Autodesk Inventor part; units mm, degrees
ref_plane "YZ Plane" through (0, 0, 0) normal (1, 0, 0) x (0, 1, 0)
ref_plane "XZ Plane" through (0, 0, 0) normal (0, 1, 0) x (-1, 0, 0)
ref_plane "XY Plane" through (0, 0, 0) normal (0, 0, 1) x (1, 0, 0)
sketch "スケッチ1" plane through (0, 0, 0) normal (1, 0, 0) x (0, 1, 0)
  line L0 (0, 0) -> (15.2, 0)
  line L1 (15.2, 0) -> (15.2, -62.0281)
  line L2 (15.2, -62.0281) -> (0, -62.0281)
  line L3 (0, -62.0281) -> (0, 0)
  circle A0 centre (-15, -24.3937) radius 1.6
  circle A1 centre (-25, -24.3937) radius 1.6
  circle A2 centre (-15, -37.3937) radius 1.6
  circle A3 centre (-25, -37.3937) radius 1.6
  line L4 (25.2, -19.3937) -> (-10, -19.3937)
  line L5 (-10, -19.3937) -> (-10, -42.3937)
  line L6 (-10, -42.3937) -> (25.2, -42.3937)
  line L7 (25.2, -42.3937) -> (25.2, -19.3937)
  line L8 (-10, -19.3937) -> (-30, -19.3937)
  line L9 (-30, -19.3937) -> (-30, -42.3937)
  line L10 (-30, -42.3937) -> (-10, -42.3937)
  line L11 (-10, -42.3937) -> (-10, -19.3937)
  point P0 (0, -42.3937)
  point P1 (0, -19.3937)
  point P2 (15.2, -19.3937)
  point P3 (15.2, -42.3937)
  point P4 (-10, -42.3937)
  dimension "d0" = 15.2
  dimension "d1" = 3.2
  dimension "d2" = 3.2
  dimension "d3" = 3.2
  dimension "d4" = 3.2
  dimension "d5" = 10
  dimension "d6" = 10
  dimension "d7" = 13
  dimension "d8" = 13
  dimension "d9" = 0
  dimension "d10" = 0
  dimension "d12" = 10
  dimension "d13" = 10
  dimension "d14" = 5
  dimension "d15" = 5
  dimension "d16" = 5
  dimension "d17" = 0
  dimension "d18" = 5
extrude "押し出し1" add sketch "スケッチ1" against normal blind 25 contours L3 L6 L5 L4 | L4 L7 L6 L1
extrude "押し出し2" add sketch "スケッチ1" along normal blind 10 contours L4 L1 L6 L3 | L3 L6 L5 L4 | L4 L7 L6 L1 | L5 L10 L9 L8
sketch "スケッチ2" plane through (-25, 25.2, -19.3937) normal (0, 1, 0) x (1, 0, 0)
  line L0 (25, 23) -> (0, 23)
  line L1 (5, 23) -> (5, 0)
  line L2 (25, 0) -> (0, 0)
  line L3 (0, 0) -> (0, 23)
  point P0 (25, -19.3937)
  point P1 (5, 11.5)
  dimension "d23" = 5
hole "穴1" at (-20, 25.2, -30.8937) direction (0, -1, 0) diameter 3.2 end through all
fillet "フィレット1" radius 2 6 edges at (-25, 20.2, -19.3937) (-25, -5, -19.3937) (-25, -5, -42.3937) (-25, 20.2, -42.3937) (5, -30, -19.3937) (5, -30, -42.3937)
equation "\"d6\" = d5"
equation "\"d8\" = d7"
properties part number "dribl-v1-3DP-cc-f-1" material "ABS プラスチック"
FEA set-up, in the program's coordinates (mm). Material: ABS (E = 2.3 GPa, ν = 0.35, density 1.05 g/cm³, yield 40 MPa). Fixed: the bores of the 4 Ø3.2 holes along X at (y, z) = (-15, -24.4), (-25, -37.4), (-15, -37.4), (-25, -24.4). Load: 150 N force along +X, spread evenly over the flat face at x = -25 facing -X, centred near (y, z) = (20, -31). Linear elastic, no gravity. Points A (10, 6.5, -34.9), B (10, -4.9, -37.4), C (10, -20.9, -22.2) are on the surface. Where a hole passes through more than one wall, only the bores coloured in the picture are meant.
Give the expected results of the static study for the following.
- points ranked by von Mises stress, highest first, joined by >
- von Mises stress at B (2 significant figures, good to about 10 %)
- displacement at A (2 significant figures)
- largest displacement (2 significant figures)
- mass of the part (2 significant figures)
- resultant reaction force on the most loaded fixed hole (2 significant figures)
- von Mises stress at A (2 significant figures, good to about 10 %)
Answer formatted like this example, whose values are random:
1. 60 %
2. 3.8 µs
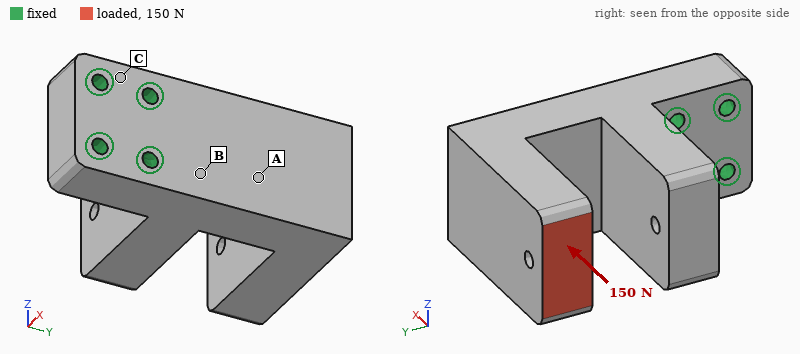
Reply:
1. B > A > C
2. 7.7 MPa
3. 0.23 mm
4. 0.79 mm
5. 25 g
6. 110 N
7. 4.8 MPa
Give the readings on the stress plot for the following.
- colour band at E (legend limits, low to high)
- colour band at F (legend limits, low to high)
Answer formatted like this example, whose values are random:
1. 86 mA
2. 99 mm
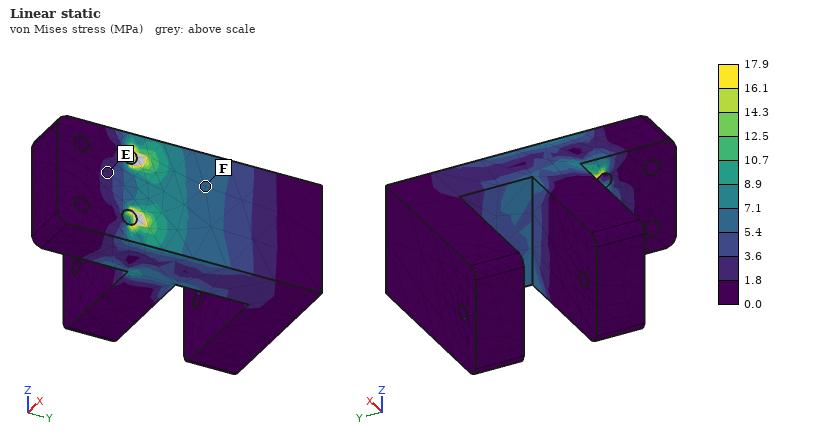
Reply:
1. 1.8 to 3.6 MPa
2. 5.4 to 7.1 MPa
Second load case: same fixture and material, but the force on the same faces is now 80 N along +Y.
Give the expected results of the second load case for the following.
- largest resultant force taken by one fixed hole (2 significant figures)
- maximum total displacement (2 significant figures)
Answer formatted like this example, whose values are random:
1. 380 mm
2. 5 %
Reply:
1. 40 N
2. 0.75 mm
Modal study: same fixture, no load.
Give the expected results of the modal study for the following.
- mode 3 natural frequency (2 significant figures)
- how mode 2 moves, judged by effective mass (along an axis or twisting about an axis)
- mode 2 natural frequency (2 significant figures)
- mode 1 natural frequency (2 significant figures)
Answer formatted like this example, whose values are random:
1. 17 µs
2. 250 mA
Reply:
1. 1900 Hz
2. along Z
3. 1200 Hz
4. 750 Hz
